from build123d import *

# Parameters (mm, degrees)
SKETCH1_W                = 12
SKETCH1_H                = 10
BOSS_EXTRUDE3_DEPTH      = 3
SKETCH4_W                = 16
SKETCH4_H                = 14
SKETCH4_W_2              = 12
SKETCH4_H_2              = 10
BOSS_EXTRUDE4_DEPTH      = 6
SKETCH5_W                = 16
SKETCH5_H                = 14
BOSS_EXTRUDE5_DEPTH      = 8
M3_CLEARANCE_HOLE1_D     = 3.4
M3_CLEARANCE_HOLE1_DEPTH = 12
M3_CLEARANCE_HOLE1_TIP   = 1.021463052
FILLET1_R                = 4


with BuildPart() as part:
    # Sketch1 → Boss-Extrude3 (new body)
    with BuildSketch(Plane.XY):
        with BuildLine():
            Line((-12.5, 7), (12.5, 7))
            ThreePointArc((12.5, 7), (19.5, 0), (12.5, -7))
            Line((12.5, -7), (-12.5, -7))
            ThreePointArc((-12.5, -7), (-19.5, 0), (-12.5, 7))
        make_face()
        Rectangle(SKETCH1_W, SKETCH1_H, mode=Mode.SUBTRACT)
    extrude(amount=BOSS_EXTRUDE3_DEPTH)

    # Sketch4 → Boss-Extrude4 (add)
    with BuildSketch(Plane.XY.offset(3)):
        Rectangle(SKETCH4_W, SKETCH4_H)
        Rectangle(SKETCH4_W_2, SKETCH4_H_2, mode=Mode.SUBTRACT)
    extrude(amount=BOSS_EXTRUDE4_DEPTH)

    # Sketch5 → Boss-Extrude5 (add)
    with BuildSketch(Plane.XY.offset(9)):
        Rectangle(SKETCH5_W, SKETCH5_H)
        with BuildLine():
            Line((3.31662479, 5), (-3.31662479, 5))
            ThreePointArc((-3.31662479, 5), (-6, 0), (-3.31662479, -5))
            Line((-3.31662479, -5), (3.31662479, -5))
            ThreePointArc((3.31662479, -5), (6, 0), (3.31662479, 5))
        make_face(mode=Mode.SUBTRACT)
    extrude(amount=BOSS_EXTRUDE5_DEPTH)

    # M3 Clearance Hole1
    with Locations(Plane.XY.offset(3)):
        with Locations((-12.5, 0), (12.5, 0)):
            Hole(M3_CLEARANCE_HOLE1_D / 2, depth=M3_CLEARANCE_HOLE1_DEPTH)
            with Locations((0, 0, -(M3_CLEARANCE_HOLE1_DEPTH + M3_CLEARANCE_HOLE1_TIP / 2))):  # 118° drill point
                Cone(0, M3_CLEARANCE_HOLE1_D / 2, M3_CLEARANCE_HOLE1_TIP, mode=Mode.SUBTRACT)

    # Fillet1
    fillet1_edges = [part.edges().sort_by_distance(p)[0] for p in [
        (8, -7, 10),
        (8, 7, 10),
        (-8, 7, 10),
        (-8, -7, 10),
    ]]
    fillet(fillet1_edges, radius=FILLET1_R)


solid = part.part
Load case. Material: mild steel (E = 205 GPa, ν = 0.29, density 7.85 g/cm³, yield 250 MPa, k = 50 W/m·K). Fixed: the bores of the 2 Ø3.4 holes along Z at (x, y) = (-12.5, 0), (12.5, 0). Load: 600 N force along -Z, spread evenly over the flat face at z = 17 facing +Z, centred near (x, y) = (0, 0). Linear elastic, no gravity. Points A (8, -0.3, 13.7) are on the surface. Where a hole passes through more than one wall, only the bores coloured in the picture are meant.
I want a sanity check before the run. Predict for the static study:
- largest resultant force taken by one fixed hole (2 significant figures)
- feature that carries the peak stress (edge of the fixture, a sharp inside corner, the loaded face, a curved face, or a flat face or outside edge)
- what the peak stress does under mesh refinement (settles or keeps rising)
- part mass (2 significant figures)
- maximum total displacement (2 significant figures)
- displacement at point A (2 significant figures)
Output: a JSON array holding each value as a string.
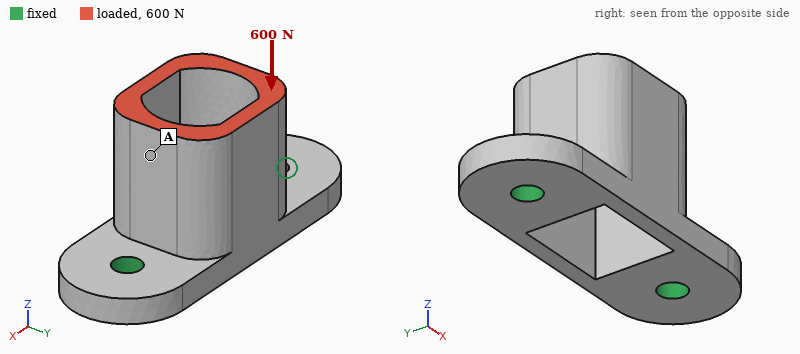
["310 N", "edge of the fixture", "keeps rising", "20 g", "2.5 µm", "2.3 µm"]
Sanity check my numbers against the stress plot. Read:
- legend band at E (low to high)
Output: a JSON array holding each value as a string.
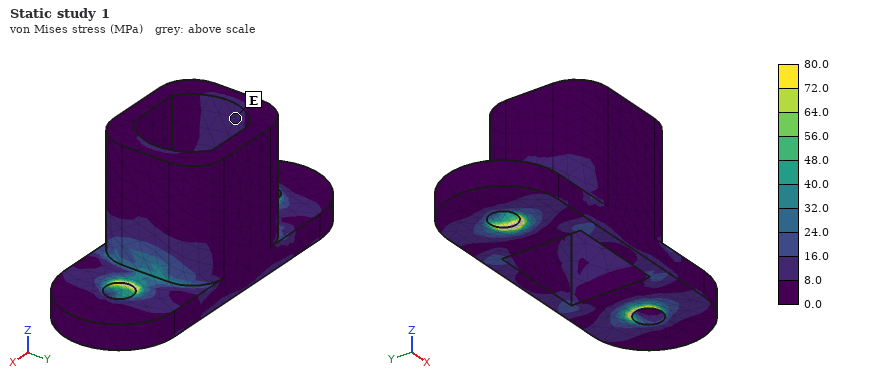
["8.0 to 16.0 MPa"]
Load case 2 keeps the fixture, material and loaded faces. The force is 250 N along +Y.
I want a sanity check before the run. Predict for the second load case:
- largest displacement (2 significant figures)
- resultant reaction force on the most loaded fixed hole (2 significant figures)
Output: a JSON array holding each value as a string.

["19 µm", "130 N"]
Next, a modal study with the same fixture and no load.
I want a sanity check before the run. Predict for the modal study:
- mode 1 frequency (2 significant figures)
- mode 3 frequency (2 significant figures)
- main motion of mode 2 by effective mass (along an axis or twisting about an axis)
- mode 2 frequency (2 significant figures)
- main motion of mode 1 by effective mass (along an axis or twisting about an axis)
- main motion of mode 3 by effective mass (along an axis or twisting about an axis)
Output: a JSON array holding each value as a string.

["8300 Hz", "22 kHz", "along X", "19 kHz", "along Y", "along Z"]
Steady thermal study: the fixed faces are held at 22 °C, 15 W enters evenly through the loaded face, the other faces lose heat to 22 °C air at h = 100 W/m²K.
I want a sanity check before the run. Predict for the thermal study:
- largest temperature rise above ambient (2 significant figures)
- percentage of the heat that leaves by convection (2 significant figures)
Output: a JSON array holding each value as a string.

["53 K", "37 %"]
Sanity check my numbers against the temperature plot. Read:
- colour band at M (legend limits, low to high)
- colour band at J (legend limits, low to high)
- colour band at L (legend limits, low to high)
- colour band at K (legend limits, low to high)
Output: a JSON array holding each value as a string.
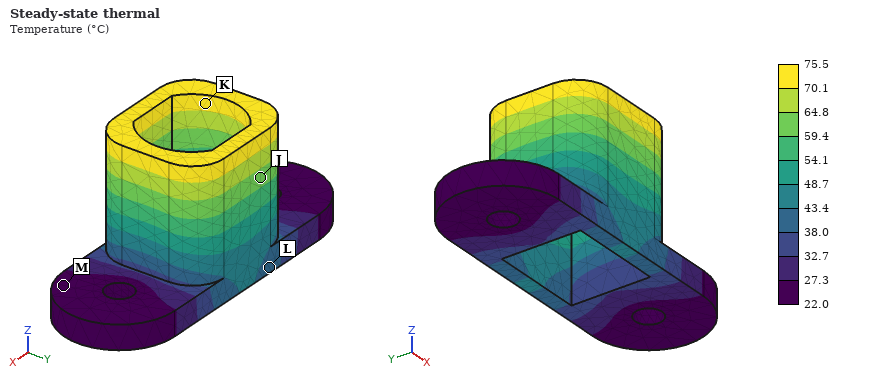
["22.0 to 27.3 °C", "59.4 to 64.8 °C", "38.0 to 43.4 °C", "70.1 to 75.5 °C"]
